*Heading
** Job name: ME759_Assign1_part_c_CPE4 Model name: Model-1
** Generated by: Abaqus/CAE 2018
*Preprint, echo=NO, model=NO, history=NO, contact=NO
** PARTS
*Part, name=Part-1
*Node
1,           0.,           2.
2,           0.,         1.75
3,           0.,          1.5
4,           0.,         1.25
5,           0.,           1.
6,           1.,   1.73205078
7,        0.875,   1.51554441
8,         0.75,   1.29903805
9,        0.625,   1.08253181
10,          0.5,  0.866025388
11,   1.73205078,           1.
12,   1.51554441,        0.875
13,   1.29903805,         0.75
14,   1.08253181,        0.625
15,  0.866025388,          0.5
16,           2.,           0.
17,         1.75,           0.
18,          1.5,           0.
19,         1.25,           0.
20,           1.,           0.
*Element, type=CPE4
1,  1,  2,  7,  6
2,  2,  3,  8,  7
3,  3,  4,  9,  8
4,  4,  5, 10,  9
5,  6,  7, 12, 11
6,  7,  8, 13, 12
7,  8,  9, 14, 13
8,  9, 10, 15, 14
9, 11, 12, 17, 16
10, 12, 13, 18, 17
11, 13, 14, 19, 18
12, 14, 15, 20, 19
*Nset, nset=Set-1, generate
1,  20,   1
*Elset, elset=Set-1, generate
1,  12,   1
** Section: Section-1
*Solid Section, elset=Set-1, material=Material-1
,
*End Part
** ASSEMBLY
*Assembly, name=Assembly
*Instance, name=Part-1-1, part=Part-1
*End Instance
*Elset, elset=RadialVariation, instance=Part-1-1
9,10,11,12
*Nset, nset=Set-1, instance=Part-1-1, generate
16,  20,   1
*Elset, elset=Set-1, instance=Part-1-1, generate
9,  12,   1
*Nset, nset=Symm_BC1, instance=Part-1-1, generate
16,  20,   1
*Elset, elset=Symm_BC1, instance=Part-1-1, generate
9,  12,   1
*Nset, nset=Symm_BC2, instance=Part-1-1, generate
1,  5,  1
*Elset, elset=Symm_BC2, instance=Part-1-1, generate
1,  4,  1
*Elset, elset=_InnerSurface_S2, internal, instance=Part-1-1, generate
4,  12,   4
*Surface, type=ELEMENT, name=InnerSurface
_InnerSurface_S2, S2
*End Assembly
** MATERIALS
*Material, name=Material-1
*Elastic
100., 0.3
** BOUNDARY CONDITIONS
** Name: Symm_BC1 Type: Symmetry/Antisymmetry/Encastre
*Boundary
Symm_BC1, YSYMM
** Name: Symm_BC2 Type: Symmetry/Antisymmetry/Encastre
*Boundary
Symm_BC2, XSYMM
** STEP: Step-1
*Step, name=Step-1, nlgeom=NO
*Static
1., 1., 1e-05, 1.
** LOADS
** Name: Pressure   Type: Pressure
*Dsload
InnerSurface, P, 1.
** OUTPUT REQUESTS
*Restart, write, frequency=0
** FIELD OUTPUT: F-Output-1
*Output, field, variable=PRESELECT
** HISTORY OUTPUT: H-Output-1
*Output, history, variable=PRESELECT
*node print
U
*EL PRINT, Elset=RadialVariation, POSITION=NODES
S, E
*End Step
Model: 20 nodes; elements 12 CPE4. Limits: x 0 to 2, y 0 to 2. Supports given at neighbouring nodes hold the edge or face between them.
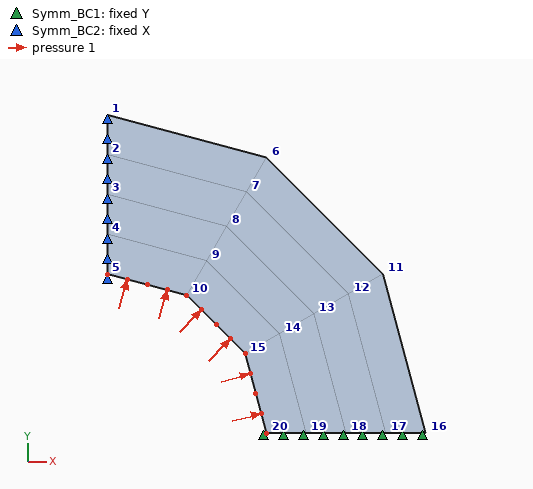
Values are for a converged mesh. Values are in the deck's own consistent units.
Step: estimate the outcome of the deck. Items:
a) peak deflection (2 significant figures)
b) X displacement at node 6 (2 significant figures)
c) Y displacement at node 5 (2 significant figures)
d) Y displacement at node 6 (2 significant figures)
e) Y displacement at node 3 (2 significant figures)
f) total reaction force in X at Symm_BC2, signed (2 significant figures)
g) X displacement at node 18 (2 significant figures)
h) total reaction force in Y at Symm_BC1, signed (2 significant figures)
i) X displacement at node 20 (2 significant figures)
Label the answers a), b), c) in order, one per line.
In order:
a) 0.019
b) 0.0059
c) 0.018
d) 0.010
e) 0.014
f) -1.0
g) 0.014
h) -1.0
i) 0.018
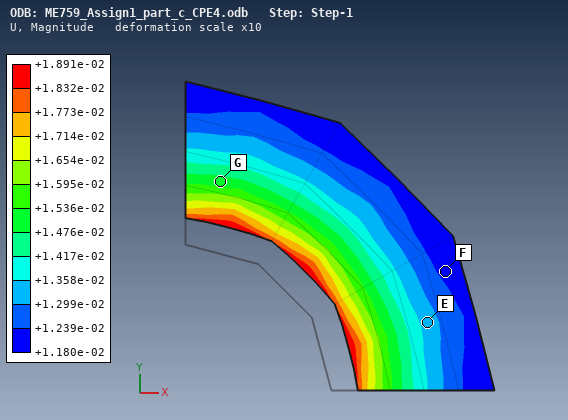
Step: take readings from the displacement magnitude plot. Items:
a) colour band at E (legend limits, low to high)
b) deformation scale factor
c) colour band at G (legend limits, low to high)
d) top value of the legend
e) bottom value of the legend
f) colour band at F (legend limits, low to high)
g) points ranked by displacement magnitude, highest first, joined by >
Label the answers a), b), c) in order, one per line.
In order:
a) +1.299e-02 to +1.358e-02
b) 10
c) +1.476e-02 to +1.536e-02
d) +1.891e-02
e) +1.180e-02
f) +1.180e-02 to +1.239e-02
g) G > E > F
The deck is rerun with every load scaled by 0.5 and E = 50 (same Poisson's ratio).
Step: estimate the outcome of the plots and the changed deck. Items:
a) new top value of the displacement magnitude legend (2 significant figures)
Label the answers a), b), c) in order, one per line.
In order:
a) 0.019
